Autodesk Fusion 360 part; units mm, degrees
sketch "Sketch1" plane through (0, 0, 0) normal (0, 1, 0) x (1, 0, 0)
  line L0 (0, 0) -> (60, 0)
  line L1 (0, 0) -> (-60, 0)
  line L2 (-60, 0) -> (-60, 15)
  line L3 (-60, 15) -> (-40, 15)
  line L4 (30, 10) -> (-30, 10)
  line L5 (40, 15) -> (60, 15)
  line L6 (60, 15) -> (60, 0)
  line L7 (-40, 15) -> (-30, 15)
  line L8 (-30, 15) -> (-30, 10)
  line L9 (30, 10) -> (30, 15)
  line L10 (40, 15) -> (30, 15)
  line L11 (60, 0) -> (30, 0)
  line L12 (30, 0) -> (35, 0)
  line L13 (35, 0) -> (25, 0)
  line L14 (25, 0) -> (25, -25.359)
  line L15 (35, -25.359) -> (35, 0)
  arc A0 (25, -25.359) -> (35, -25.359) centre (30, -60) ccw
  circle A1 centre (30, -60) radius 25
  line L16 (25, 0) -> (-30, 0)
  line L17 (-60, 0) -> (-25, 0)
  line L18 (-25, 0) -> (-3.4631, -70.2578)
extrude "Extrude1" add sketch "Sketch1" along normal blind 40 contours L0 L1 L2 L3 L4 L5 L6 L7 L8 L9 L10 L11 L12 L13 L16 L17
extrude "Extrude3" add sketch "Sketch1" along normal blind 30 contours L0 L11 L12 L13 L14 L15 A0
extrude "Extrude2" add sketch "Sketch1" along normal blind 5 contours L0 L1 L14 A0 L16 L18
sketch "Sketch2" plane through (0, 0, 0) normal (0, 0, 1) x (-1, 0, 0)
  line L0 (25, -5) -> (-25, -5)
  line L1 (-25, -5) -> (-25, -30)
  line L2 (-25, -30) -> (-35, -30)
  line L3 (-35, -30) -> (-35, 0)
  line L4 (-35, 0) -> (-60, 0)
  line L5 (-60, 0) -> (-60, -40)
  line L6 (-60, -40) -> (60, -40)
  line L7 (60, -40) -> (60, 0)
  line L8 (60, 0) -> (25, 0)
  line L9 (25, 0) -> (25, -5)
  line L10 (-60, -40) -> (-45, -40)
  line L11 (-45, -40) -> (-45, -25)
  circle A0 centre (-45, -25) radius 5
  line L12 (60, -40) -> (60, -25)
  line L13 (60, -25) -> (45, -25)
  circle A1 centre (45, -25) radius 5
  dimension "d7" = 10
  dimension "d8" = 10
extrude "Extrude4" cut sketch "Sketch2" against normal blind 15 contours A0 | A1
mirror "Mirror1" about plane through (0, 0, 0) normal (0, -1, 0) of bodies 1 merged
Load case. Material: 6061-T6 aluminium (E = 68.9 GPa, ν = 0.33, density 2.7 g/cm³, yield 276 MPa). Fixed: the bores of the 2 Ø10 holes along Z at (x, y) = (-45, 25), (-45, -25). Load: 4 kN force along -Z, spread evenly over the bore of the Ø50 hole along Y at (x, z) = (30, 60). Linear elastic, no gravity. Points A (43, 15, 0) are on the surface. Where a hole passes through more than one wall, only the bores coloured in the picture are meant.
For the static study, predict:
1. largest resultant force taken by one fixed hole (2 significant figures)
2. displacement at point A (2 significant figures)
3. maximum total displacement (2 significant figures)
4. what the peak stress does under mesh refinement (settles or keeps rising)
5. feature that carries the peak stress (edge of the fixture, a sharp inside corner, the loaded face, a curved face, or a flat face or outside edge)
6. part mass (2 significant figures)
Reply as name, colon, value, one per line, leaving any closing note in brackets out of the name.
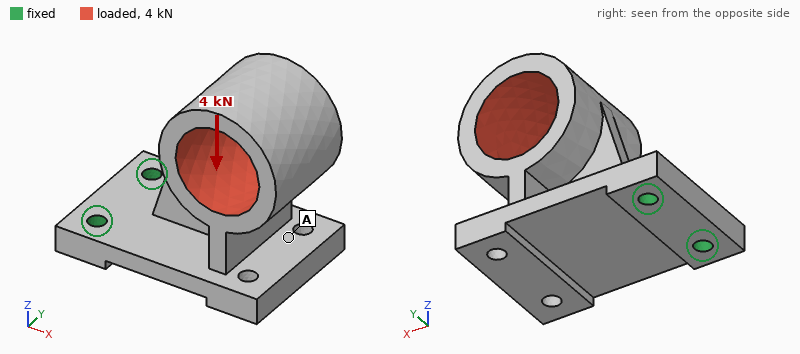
largest resultant force taken by one fixed hole: 2.0 kN
displacement at point A: 0.84 mm
maximum total displacement: 1.5 mm
what the peak stress does under mesh refinement: keeps rising
feature that carries the peak stress: edge of the fixture
part mass: 700 g
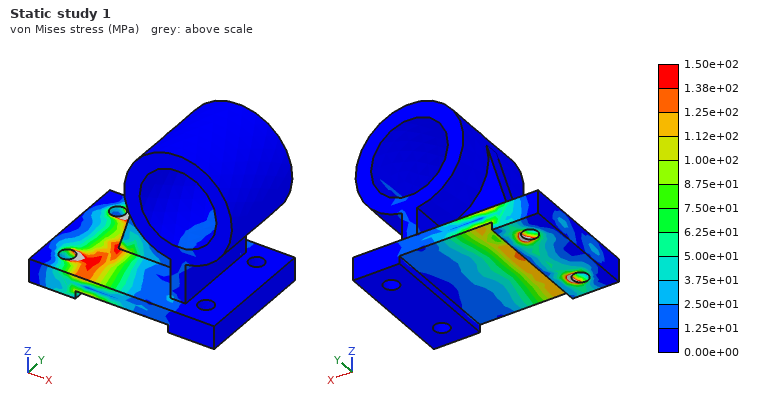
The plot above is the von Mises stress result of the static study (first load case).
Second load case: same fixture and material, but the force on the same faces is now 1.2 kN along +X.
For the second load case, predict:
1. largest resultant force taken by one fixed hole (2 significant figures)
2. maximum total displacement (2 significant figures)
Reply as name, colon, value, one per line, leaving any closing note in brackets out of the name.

largest resultant force taken by one fixed hole: 660 N
maximum total displacement: 0.52 mm
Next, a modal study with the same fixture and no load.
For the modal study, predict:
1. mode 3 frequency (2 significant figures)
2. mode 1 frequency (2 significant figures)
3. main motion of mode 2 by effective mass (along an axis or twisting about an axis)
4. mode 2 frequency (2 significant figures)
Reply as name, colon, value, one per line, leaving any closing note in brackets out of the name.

mode 3 frequency: 2300 Hz
mode 1 frequency: 380 Hz
main motion of mode 2 by effective mass: along Y
mode 2 frequency: 590 Hz
